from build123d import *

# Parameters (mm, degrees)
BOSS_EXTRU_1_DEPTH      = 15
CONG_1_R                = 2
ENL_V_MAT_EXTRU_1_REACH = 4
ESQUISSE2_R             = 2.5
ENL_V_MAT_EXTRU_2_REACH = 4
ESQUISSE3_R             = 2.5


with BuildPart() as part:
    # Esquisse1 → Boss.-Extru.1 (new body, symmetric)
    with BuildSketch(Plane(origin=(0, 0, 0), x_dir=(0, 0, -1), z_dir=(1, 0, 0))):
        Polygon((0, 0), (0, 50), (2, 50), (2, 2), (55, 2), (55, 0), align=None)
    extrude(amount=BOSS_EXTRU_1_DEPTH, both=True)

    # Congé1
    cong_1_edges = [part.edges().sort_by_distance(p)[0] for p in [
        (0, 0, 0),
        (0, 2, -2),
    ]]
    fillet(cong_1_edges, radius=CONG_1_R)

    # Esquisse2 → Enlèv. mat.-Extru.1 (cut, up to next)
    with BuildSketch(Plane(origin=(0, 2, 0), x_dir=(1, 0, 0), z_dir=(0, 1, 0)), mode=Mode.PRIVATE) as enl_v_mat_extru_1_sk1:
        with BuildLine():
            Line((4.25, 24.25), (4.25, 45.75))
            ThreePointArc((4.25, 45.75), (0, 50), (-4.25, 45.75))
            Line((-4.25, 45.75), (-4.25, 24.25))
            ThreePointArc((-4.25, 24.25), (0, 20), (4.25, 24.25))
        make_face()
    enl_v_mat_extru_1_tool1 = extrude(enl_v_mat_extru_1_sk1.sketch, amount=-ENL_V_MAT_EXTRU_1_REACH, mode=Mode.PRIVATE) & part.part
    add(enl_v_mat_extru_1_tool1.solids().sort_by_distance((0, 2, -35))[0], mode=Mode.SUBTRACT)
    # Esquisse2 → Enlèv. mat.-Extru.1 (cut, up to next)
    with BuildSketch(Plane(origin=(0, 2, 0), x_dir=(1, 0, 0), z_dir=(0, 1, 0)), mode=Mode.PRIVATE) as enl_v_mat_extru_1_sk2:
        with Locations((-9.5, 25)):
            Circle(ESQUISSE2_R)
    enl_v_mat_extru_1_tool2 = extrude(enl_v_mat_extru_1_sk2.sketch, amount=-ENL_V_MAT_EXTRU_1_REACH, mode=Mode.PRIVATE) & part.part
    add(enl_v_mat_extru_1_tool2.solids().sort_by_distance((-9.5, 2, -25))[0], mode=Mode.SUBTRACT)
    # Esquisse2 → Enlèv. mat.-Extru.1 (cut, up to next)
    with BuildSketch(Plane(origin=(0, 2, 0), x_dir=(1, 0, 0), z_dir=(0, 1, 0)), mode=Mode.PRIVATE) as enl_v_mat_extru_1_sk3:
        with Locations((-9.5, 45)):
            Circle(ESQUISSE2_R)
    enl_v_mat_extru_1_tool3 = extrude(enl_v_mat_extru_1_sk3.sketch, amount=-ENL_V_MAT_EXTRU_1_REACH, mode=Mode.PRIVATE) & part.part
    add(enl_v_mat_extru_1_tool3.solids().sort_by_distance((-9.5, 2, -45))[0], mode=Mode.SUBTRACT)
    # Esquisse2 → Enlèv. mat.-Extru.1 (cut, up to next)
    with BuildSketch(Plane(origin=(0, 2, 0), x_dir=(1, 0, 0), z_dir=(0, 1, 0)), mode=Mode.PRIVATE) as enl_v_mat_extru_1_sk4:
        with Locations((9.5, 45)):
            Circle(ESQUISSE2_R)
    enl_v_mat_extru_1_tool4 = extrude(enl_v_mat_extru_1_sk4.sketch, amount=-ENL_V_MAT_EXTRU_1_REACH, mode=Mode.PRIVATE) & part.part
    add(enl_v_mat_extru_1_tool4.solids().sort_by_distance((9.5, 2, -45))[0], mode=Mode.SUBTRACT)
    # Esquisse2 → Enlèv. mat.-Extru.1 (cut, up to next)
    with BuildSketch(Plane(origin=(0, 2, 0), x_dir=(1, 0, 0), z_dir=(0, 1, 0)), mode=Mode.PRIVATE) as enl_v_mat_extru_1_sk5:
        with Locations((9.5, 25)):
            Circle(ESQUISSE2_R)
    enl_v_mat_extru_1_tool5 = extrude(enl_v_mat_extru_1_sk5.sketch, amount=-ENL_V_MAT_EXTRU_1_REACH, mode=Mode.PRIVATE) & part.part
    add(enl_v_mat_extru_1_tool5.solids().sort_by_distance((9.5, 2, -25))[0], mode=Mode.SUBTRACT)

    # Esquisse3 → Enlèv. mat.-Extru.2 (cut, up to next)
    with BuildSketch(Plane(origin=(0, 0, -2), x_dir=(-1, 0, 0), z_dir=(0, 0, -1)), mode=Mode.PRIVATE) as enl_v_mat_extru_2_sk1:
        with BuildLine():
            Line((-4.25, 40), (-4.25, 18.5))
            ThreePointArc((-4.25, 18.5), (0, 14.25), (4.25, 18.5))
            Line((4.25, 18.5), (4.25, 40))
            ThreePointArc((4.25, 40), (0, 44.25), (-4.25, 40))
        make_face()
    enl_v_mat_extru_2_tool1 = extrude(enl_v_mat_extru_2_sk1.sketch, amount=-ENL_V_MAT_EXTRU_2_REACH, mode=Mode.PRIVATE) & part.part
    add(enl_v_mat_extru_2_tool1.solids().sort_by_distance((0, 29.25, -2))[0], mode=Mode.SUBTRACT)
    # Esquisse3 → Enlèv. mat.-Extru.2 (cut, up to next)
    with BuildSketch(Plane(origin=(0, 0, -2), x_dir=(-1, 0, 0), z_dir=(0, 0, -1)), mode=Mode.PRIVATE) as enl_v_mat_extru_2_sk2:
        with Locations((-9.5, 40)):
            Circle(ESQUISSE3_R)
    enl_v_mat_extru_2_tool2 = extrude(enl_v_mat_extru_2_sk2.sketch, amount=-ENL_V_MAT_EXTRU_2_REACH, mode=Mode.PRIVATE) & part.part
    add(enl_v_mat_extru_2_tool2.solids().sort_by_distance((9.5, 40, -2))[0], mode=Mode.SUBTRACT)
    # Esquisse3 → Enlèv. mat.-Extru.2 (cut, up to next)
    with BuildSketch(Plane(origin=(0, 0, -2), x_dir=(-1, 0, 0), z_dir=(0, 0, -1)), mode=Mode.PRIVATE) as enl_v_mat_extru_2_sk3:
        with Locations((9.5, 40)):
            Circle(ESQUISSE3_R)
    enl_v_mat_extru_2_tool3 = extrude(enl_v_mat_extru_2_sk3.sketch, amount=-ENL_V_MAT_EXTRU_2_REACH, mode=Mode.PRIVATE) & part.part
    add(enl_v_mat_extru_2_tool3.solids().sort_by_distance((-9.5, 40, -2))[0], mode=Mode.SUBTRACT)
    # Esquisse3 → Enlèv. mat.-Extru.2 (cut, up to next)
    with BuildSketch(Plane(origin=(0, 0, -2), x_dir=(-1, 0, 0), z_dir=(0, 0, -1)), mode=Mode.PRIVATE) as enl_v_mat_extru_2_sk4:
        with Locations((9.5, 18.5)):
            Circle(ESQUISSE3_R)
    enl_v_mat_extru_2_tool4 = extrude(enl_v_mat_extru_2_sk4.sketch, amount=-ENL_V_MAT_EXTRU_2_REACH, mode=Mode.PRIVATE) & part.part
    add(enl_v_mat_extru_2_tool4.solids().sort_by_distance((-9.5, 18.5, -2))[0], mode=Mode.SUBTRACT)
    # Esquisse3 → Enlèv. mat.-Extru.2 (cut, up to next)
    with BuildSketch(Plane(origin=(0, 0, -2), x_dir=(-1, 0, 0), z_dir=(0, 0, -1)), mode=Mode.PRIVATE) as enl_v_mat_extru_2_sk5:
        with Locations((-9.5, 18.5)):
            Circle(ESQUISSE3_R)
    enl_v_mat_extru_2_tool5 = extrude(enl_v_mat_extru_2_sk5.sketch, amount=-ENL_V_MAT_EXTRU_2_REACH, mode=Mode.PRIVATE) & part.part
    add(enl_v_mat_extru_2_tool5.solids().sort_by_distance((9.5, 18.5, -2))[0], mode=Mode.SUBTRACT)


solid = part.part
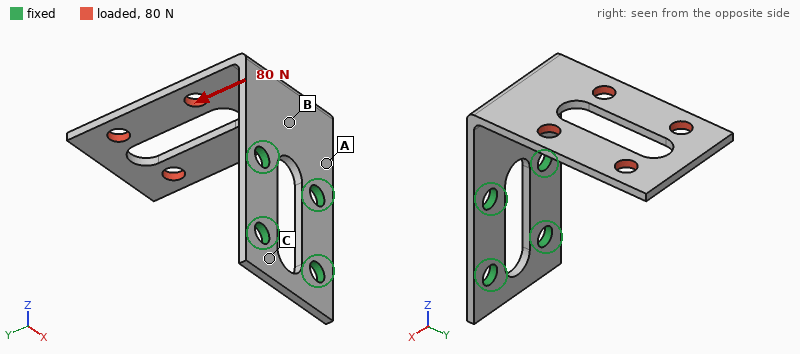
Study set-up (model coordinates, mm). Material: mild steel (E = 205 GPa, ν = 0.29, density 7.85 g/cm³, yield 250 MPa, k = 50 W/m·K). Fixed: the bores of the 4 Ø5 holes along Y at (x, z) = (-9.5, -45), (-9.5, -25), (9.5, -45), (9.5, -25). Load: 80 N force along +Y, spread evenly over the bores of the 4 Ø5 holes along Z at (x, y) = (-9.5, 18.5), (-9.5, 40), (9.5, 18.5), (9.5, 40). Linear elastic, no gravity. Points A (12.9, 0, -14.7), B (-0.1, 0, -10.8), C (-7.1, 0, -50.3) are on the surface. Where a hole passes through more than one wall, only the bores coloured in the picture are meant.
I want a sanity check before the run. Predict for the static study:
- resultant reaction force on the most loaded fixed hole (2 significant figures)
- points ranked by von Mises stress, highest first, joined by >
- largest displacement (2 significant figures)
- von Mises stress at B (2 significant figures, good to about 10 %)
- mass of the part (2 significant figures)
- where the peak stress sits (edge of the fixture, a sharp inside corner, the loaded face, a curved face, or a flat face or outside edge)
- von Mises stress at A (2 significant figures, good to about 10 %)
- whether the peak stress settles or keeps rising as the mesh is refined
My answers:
40 N
A > B > C
0.27 mm
35 MPa
39 g
edge of the fixture
60 MPa
keeps rising
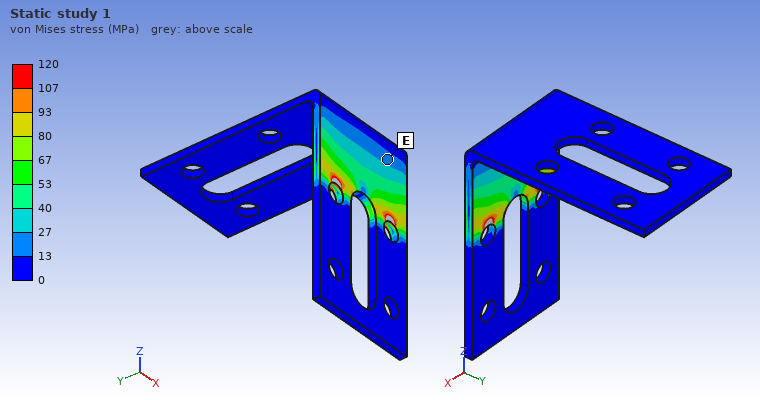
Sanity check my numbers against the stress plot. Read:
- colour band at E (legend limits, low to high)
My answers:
13 to 27 MPa
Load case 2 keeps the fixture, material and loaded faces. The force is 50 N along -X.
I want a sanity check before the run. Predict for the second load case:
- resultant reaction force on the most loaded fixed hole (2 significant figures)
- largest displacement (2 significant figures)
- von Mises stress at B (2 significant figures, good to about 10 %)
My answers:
81 N
0.14 mm
41 MPa
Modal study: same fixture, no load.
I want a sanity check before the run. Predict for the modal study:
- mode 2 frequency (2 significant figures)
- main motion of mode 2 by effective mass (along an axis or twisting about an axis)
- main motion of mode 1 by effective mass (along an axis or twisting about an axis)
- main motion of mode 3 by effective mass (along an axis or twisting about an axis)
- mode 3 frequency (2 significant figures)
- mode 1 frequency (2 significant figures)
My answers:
900 Hz
along X
along Z
along Y
1500 Hz
440 Hz
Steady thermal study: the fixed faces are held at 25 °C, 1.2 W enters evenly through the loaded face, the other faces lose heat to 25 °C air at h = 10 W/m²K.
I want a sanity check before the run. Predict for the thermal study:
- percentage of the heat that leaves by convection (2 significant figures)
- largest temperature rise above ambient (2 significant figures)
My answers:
33 %
18 K
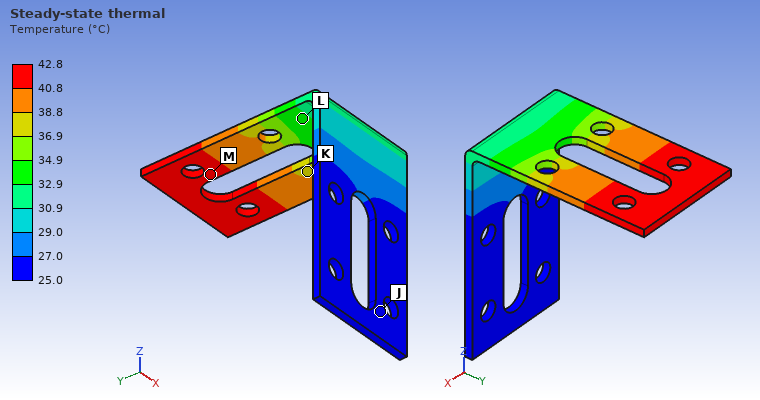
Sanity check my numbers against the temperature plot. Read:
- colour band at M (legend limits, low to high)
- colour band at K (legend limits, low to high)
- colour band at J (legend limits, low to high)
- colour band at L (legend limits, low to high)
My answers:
40.8 to 42.8 °C
36.9 to 38.8 °C
25.0 to 27.0 °C
32.9 to 34.9 °C
